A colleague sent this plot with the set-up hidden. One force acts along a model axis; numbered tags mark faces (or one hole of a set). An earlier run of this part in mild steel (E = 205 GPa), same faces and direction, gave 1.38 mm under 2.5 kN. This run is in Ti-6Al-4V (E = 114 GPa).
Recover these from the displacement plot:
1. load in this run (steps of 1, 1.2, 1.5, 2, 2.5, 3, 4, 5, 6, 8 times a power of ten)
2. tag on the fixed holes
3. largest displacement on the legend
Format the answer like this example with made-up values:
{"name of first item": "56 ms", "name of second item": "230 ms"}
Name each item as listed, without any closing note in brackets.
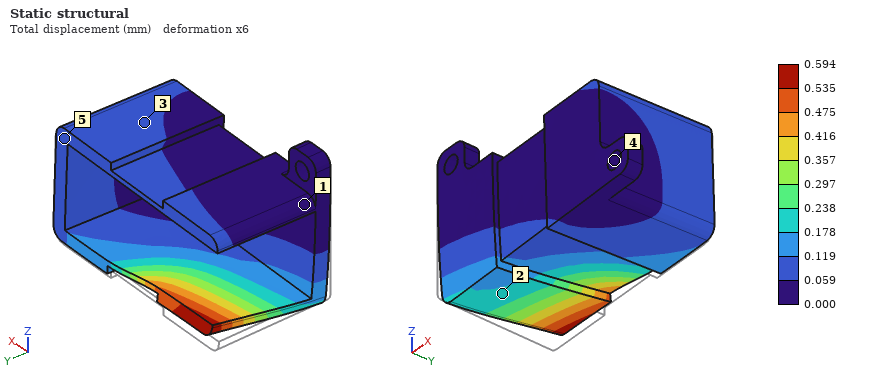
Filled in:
{"load in this run": "600 N", "tag on the fixed holes": "4", "largest displacement on the legend": "0.594 mm"}
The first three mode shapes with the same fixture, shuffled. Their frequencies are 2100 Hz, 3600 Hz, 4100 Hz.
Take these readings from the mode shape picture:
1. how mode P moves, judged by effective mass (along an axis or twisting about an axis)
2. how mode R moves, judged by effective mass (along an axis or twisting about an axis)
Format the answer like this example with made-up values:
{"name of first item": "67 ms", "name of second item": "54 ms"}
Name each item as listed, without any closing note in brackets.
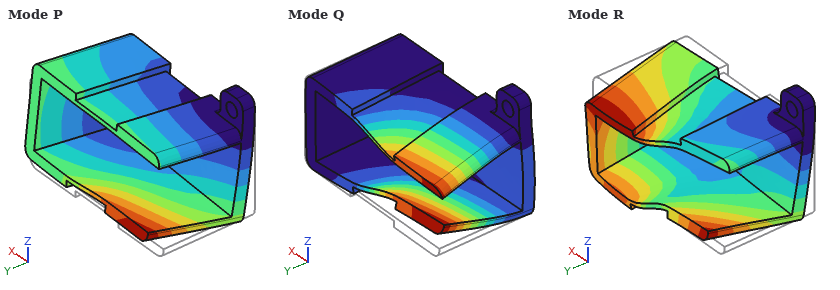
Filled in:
{"how mode P moves, judged by effective mass": "along Z", "how mode R moves, judged by effective mass": "along Y"}
